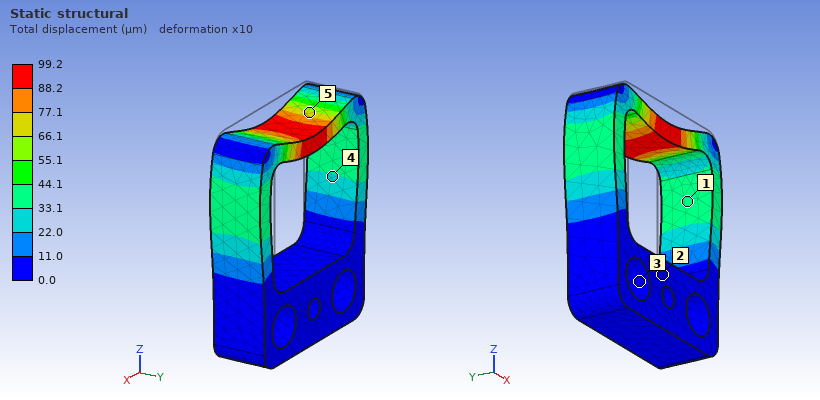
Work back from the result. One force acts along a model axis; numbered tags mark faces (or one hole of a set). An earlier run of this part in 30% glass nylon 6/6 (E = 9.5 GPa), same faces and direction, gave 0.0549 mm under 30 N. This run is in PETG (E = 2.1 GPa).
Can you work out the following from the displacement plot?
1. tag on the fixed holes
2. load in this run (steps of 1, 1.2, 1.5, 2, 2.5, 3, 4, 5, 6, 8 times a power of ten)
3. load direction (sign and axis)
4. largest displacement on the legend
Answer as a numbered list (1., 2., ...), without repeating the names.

1. 3
2. 12 N
3. -Z
4. 99.2 µm
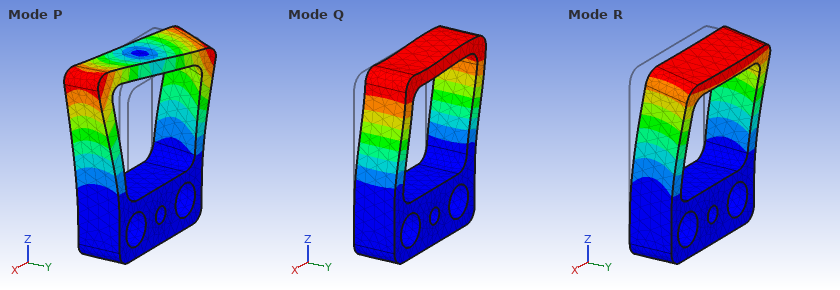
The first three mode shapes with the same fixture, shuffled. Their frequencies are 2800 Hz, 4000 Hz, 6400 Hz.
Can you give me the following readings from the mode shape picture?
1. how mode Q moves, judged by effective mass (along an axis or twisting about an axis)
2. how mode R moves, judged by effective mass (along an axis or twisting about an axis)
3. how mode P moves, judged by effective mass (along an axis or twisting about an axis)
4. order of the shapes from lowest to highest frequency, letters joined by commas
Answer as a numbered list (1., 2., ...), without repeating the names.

1. along X
2. along Y
3. twisting about Z
4. Q, R, P
